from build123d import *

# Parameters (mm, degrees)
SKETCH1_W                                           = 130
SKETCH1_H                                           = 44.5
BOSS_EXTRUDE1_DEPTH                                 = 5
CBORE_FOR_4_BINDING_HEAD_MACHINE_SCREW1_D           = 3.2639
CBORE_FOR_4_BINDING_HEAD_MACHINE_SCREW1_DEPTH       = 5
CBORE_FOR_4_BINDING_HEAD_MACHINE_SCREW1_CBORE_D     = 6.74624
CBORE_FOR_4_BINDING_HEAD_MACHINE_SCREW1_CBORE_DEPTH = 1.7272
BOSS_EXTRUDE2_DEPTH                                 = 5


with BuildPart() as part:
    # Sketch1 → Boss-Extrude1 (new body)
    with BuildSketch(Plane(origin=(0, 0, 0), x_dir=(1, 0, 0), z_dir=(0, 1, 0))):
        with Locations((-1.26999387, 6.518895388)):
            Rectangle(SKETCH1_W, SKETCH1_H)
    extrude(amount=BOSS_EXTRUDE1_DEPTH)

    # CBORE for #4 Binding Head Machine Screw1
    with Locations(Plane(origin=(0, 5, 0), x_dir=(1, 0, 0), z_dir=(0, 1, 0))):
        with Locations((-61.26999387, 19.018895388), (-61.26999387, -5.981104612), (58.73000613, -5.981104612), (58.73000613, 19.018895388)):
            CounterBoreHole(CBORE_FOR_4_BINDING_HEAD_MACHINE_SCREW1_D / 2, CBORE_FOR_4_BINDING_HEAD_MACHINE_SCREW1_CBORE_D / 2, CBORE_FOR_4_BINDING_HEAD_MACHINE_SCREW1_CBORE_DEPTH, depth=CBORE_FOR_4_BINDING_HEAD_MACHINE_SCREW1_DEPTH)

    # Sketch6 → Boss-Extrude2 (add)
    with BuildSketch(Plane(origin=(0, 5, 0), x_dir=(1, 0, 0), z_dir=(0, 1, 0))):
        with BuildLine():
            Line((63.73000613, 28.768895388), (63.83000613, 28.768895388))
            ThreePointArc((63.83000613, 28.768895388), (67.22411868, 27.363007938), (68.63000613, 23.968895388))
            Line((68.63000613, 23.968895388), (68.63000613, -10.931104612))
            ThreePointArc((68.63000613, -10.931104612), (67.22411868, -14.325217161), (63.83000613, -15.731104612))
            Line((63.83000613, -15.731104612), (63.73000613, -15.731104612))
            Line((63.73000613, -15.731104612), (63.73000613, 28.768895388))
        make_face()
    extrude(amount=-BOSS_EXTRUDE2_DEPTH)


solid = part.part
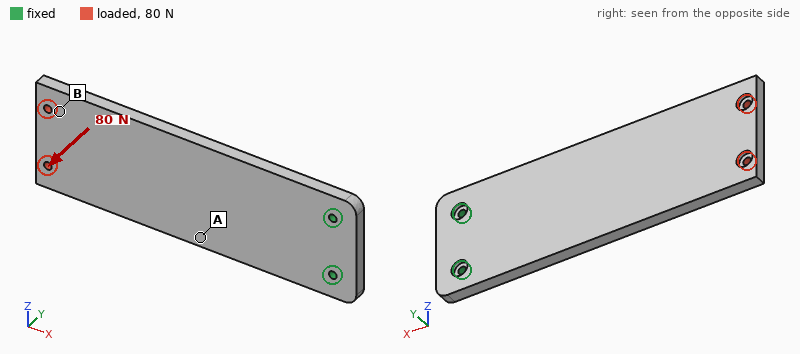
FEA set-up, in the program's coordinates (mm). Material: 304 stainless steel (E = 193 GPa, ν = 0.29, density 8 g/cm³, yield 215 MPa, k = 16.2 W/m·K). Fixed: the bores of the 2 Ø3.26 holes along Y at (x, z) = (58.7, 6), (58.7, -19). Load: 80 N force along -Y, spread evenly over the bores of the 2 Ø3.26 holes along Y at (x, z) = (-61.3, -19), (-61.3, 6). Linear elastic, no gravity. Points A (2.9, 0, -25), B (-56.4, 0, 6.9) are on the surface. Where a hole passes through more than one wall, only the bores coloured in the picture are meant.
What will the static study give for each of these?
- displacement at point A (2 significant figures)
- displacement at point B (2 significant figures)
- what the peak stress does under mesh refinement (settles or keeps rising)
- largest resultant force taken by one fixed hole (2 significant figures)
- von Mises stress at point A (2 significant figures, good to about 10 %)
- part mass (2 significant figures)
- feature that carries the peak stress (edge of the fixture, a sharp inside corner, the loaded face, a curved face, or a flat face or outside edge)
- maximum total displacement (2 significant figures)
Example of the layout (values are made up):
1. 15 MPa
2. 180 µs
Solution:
1. 0.18 mm
2. 0.57 mm
3. keeps rising
4. 90 N
5. 28 MPa
6. 240 g
7. edge of the fixture
8. 0.64 mm
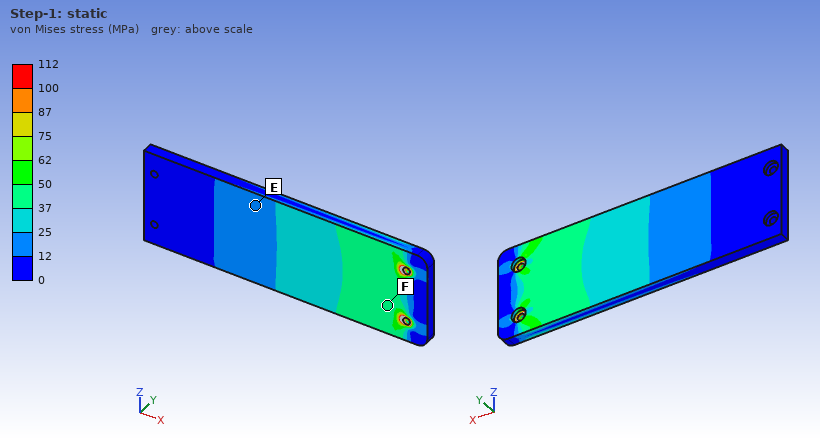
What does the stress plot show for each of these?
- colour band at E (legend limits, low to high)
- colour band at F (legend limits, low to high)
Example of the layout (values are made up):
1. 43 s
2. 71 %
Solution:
1. 12 to 25 MPa
2. 37 to 50 MPa
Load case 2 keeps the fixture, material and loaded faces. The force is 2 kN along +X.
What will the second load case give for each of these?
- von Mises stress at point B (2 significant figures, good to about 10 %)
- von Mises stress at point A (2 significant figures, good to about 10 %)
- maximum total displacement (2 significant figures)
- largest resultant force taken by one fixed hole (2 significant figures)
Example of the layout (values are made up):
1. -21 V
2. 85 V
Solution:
1. 29 MPa
2. 18 MPa
3. 0.14 mm
4. 1.0 kN
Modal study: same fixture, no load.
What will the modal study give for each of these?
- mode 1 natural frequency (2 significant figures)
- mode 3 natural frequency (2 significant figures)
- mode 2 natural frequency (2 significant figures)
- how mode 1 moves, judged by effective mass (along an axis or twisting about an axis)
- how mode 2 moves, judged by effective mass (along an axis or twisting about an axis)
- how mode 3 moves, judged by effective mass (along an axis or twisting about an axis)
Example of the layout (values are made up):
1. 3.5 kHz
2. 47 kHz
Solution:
1. 230 Hz
2. 1500 Hz
3. 1400 Hz
4. along Y
5. twisting about X
6. along Y
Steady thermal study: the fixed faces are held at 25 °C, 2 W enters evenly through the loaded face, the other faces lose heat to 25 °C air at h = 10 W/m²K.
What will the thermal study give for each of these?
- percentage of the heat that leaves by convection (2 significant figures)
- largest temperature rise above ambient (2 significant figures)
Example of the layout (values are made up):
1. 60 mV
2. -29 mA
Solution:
1. 78 %
2. 33 K
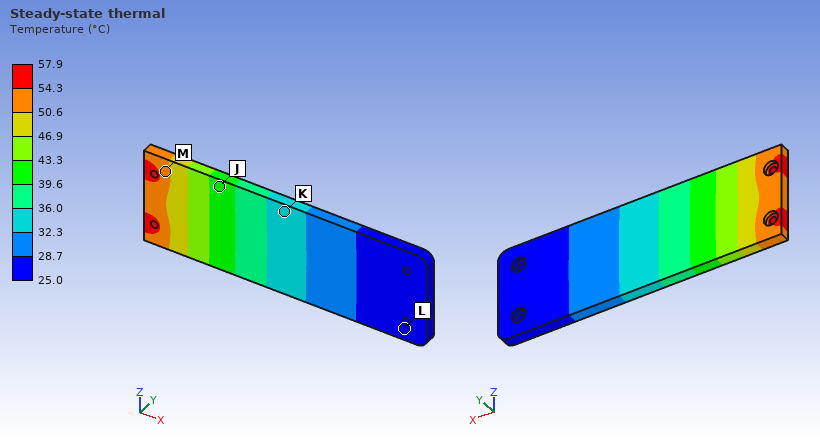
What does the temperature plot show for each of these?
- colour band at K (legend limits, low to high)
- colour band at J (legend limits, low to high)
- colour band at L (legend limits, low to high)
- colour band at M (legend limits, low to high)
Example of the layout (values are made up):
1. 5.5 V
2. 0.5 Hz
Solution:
1. 32.3 to 36.0 °C
2. 39.6 to 43.3 °C
3. 25.0 to 28.7 °C
4. 50.6 to 54.3 °C
